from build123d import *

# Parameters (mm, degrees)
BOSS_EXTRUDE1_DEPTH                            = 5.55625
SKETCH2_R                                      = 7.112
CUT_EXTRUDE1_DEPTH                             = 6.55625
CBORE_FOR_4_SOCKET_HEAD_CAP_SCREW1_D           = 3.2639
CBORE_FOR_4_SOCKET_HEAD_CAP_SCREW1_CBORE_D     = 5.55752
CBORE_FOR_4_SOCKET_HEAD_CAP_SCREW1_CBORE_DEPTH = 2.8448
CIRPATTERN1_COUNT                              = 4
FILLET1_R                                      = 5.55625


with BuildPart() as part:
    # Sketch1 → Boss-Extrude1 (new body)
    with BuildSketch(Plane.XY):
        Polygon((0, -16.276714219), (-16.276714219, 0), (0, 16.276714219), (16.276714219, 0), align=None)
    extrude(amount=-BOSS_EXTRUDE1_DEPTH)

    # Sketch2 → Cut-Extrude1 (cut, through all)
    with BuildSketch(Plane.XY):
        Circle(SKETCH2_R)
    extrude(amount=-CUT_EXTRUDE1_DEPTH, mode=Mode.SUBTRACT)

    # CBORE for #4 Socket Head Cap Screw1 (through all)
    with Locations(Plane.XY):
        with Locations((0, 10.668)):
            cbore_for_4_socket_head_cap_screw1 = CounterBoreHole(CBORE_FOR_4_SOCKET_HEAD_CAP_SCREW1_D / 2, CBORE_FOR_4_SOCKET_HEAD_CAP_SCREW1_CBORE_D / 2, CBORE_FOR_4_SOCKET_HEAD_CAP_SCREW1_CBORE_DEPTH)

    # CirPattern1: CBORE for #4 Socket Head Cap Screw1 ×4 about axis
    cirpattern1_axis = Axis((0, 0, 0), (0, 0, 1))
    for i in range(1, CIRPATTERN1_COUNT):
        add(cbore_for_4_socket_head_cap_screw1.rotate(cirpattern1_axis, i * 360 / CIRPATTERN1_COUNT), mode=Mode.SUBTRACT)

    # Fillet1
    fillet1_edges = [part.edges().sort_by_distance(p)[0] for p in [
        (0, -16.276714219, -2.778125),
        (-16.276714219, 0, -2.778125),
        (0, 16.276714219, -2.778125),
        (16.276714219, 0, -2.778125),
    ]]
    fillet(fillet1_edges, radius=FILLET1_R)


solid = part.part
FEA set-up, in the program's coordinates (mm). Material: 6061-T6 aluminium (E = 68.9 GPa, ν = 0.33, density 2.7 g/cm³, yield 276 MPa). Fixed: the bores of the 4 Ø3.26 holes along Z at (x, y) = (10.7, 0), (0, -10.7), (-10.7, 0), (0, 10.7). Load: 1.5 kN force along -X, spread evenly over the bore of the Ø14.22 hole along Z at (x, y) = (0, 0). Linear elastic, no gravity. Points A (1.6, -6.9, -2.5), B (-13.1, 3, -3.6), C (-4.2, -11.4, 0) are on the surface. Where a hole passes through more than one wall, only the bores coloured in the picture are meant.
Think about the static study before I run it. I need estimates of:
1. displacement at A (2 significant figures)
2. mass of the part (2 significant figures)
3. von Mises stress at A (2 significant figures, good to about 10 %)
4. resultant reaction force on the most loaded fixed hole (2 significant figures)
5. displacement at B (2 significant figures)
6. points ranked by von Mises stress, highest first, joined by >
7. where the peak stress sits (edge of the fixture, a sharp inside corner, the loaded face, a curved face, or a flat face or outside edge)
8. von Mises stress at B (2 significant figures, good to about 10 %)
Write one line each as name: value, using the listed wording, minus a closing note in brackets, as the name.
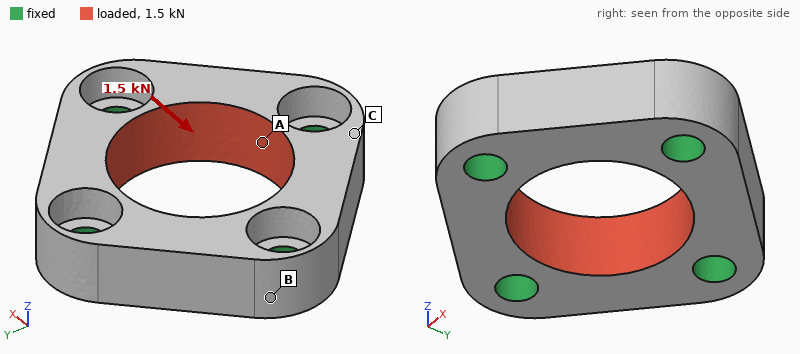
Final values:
displacement at A: 1.8 µm
mass of the part: 4.2 g
von Mises stress at A: 17 MPa
resultant reaction force on the most loaded fixed hole: 380 N
displacement at B: 0.92 µm
points ranked by von Mises stress, highest first, joined by >: A > B > C
where the peak stress sits: edge of the fixture
von Mises stress at B: 12 MPa
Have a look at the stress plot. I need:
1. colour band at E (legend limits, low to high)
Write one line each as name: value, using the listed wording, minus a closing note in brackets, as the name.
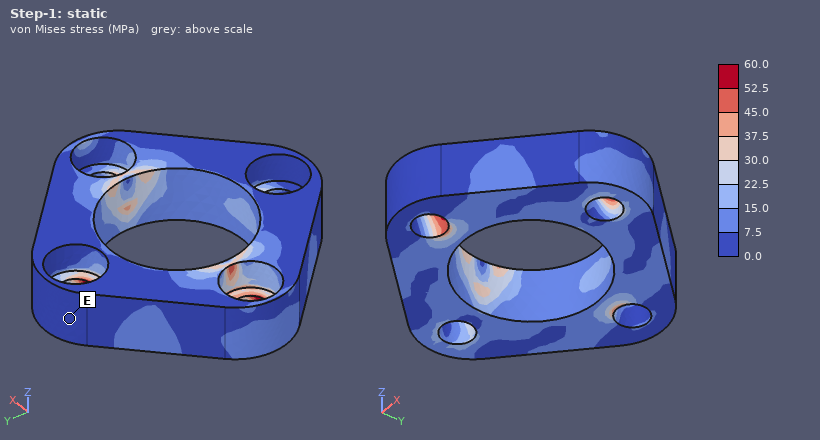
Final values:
colour band at E: 0.0 to 7.5 MPa
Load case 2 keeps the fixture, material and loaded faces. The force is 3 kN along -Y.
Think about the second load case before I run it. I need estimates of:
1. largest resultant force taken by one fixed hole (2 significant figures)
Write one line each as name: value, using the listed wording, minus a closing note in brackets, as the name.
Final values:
largest resultant force taken by one fixed hole: 760 N
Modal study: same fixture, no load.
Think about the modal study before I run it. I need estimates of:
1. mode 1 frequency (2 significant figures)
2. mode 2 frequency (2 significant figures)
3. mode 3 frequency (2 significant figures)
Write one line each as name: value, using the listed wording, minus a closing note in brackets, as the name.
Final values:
mode 1 frequency: 54 kHz
mode 2 frequency: 62 kHz
mode 3 frequency: 62 kHz
